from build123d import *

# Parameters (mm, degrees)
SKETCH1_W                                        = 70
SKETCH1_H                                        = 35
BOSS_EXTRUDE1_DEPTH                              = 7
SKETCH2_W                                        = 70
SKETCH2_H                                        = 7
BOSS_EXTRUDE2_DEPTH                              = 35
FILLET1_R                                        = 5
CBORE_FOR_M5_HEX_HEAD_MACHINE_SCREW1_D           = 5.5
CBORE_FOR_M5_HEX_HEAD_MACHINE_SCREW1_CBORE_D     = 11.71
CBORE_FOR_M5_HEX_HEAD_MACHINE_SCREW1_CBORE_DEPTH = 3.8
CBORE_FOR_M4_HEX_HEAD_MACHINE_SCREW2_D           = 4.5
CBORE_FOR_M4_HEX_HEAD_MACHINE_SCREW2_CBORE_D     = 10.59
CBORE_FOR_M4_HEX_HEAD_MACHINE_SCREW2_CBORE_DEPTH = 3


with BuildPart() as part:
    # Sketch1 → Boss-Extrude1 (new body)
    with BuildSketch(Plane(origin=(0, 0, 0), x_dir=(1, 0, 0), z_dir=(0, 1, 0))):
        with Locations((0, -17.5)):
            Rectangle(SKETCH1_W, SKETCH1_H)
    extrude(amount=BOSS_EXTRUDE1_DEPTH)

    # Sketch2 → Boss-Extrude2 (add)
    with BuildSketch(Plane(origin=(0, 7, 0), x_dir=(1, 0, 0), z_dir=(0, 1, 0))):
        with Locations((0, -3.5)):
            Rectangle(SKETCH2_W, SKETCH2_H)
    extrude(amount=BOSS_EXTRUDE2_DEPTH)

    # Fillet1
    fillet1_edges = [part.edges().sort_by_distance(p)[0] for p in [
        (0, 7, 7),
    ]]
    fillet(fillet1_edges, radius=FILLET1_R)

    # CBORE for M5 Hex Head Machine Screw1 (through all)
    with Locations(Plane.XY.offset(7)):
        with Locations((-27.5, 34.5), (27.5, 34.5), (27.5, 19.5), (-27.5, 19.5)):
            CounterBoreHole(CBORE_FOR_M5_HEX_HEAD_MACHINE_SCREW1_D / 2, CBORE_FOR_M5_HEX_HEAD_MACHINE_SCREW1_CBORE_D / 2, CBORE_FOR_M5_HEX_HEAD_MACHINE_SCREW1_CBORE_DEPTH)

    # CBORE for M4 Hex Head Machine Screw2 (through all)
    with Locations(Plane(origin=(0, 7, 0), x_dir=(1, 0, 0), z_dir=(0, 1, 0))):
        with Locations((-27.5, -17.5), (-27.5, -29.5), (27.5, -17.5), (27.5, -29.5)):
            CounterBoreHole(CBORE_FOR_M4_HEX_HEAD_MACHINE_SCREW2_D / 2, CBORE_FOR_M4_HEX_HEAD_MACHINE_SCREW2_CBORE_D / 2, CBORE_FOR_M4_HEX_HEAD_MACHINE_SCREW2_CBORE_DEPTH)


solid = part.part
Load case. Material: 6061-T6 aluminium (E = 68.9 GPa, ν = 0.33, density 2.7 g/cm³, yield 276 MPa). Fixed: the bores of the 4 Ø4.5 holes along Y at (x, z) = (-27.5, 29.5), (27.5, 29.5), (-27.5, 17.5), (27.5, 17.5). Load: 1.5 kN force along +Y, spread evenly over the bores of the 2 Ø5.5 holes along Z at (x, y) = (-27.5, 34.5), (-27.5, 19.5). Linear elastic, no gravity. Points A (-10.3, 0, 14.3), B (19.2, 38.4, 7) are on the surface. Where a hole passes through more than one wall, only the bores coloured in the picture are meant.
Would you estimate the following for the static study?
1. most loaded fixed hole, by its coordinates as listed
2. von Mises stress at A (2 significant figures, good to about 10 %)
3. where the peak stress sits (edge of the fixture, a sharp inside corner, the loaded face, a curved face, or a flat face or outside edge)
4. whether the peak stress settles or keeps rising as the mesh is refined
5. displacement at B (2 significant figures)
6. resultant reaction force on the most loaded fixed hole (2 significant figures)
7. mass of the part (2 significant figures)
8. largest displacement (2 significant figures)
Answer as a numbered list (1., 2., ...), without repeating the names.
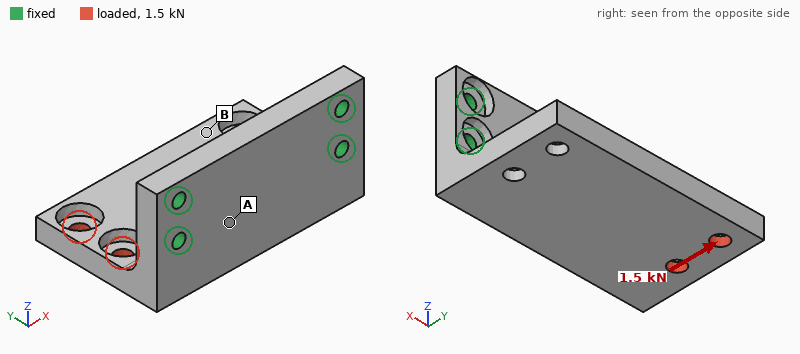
1. (-27.5, 17.5)
2. 27 MPa
3. edge of the fixture
4. keeps rising
5. 0.084 mm
6. 2.2 kN
7. 85 g
8. 0.18 mm
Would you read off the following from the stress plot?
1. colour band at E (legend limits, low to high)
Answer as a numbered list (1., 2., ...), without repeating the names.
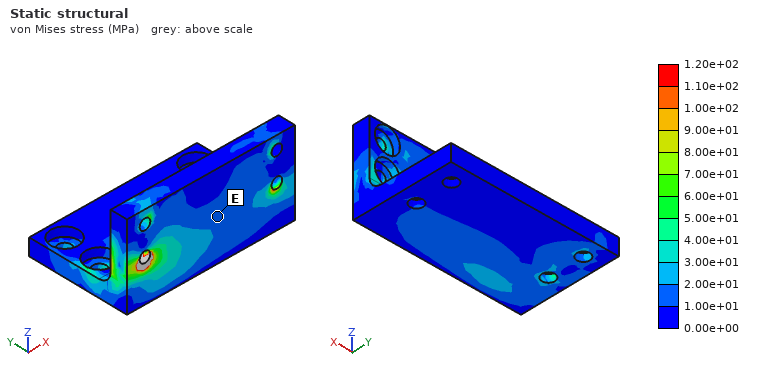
1. 1.00e+01 to 2.00e+01 MPa
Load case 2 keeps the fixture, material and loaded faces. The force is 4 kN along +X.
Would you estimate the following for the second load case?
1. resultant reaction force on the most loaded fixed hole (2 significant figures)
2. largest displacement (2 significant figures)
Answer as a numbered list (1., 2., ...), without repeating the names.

1. 2.7 kN
2. 96 µm
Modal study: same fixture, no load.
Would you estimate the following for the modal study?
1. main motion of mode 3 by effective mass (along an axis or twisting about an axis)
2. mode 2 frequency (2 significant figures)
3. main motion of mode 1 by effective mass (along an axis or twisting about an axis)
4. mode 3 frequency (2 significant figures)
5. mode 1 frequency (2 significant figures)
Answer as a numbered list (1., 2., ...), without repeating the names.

1. along Y
2. 4600 Hz
3. along Z
4. 6900 Hz
5. 2200 Hz
